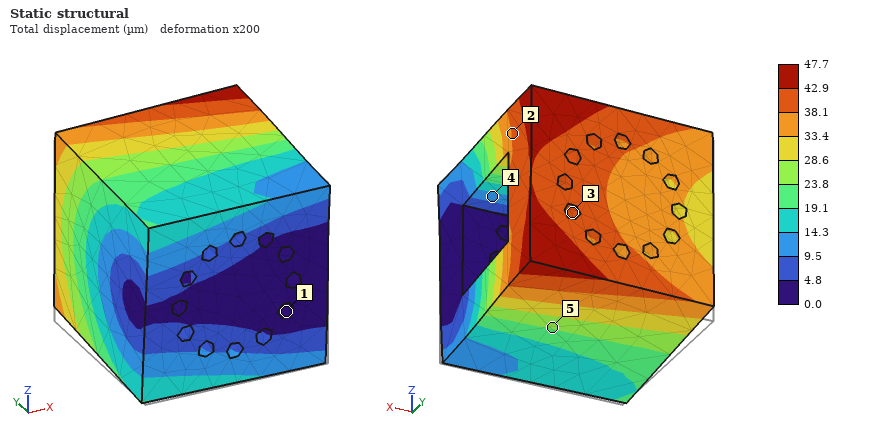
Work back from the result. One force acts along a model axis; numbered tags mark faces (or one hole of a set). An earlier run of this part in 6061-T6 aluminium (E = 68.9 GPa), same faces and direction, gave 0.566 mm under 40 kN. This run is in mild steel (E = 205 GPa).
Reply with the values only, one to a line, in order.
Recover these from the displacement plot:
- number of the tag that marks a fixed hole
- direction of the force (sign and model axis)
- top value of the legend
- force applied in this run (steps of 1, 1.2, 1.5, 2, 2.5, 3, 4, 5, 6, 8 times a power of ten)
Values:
1
+Z
47.7 µm
10 kN
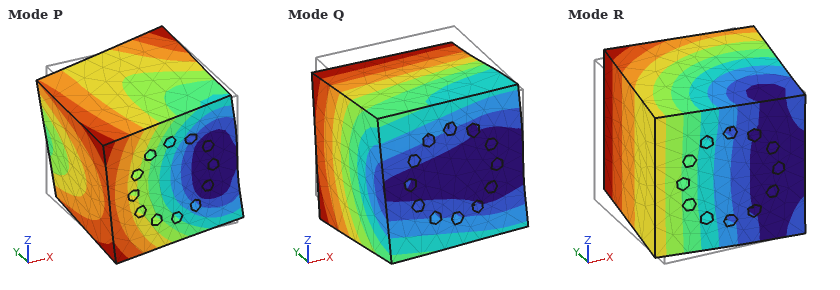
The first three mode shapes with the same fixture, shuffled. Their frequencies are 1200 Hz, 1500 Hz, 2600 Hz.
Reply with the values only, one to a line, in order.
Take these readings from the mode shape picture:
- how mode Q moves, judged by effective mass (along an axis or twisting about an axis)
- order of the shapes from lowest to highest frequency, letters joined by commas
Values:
along Z
R, Q, P
